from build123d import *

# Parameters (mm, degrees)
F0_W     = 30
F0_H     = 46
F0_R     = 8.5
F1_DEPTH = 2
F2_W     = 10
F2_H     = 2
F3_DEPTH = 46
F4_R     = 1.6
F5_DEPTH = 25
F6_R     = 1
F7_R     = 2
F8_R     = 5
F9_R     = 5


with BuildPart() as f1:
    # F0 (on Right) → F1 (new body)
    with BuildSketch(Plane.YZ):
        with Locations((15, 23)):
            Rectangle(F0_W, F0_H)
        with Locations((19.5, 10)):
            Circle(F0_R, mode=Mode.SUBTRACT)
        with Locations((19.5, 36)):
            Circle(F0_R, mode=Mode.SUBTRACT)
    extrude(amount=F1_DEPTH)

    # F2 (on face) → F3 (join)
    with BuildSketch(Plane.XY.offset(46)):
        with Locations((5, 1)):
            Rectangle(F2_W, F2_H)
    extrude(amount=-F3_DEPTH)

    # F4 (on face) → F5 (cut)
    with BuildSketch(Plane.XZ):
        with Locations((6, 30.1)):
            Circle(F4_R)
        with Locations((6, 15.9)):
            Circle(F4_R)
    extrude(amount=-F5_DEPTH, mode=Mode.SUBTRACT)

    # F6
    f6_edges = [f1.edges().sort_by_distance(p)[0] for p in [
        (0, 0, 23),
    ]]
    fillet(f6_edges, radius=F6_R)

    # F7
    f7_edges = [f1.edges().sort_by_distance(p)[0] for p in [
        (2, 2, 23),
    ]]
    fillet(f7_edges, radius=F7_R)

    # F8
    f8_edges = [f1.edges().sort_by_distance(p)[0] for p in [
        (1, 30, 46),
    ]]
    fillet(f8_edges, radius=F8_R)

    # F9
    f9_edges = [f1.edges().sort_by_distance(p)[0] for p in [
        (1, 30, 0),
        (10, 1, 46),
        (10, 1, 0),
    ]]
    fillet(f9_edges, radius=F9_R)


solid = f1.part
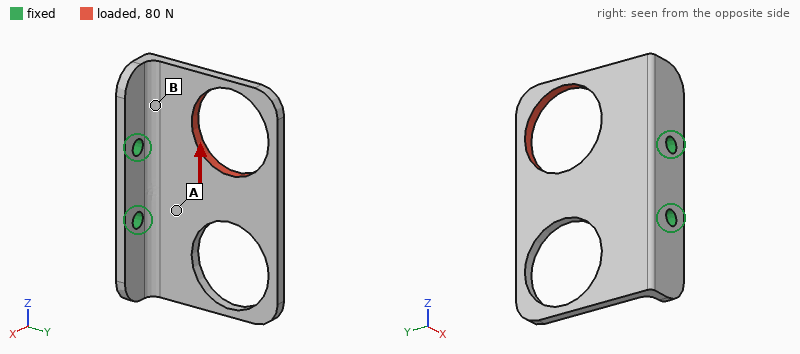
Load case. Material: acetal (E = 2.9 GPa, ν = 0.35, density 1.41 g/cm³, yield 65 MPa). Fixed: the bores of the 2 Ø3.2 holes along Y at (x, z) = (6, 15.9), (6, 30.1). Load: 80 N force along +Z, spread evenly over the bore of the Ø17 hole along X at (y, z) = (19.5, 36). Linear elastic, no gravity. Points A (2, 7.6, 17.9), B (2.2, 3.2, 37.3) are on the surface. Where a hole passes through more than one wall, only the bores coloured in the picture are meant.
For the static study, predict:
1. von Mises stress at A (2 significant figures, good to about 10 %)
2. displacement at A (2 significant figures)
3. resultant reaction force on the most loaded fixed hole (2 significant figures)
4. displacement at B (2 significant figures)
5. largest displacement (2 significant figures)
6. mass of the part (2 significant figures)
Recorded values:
9.2 MPa
0.11 mm
100 N
0.14 mm
0.64 mm
3.6 g
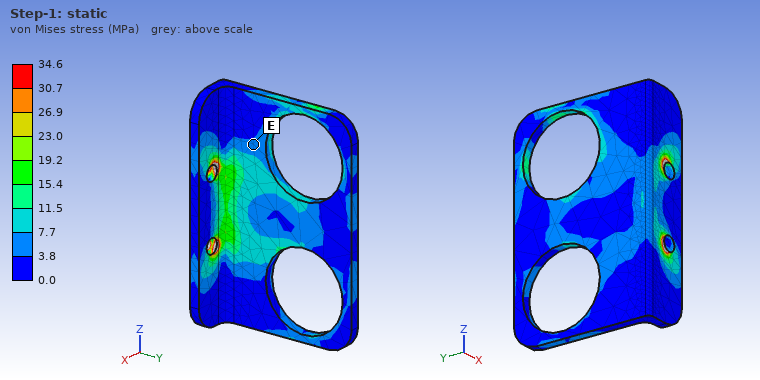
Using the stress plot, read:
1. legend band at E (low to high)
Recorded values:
3.8 to 7.7 MPa
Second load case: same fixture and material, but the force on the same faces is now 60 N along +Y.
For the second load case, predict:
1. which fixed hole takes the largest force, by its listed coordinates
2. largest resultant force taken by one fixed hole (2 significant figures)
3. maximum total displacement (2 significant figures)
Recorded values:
(6, 30.1)
77 N
0.57 mm
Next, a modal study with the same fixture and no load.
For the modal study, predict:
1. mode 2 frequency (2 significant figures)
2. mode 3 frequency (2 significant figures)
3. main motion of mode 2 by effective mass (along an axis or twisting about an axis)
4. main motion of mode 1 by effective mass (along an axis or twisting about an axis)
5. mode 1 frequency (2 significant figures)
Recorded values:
930 Hz
1700 Hz
twisting about Y
along X
540 Hz
